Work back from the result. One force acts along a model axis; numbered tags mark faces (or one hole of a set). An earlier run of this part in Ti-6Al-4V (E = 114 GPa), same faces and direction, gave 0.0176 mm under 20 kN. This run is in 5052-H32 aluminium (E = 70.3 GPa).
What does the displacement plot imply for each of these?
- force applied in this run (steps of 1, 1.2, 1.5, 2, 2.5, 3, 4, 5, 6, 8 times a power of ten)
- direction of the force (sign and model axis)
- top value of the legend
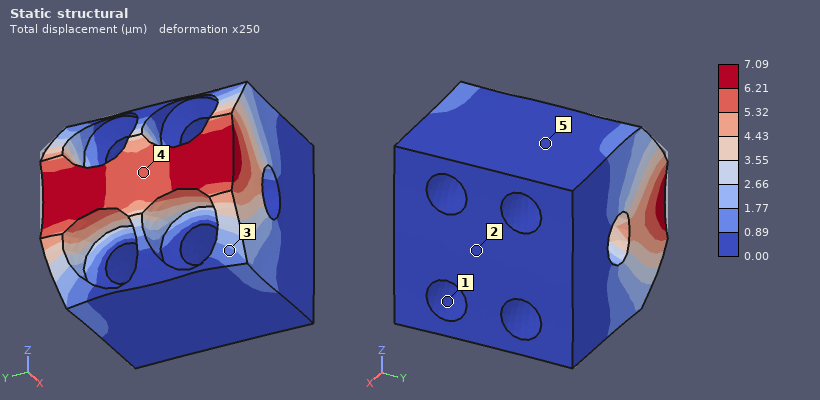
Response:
5 kN
+X
7.09 µm
